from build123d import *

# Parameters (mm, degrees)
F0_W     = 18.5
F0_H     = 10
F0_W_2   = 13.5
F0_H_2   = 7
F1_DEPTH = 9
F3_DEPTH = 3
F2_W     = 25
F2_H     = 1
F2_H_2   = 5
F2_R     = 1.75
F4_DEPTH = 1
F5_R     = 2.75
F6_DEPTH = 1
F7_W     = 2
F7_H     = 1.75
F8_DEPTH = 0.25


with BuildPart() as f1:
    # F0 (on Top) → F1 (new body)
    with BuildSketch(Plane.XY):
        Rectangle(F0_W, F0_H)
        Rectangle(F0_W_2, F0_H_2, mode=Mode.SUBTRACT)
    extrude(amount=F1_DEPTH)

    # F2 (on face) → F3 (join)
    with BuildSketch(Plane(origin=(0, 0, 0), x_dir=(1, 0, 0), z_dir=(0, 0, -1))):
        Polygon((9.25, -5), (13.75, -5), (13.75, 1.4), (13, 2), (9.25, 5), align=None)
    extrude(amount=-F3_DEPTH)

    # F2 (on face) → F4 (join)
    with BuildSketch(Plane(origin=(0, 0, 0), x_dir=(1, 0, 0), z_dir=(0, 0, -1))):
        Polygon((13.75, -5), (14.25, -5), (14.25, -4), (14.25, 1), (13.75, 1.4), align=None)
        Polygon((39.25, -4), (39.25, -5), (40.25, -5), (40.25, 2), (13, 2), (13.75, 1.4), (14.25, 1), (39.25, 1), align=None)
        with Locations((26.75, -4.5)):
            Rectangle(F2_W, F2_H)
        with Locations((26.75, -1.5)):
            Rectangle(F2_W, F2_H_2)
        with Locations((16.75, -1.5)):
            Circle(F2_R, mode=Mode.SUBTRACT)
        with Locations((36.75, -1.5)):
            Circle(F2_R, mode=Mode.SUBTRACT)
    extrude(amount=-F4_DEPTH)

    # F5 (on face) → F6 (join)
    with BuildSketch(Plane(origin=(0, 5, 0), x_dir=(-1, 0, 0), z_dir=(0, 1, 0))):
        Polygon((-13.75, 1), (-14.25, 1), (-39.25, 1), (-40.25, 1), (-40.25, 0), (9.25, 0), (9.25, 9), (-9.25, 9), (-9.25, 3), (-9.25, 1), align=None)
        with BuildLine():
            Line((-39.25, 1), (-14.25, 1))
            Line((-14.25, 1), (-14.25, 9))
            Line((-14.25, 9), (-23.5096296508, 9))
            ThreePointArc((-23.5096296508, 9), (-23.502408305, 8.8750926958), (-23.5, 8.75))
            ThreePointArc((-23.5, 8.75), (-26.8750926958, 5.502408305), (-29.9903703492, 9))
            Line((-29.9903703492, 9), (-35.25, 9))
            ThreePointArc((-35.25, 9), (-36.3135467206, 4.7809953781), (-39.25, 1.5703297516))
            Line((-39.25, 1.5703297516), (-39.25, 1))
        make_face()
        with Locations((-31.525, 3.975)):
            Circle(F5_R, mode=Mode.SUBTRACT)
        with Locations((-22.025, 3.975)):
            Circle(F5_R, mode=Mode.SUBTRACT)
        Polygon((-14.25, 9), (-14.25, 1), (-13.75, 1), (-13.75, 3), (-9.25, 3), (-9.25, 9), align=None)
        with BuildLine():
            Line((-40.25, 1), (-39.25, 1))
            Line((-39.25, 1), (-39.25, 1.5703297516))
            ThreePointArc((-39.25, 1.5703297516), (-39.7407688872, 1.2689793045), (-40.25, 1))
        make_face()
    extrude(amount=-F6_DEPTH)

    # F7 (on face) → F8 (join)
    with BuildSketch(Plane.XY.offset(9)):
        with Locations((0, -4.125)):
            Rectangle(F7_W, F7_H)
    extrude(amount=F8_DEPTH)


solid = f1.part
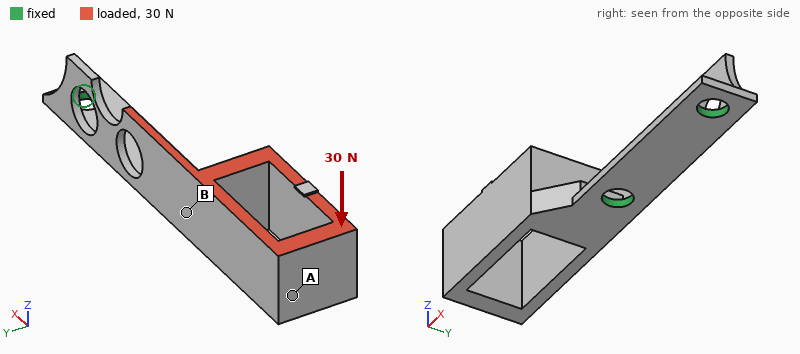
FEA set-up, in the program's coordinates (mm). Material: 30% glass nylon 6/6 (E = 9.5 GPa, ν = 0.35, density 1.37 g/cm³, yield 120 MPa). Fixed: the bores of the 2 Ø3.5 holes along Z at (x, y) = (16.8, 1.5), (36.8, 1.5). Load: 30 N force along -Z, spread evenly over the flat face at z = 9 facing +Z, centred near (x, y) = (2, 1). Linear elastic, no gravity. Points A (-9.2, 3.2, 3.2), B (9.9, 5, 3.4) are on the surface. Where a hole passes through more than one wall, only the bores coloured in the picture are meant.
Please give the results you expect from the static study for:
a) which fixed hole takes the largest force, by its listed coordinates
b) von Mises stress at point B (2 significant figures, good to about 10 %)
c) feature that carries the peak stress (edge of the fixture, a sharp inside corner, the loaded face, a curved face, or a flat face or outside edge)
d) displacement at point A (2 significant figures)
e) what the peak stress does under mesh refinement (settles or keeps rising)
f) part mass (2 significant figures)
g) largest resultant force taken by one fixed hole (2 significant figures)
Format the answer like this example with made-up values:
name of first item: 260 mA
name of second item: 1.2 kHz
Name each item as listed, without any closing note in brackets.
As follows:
which fixed hole takes the largest force, by its listed coordinates: (16.8, 1.5)
von Mises stress at point B: 7.5 MPa
feature that carries the peak stress: edge of the fixture
displacement at point A: 0.33 mm
what the peak stress does under mesh refinement: keeps rising
part mass: 1.7 g
largest resultant force taken by one fixed hole: 48 N
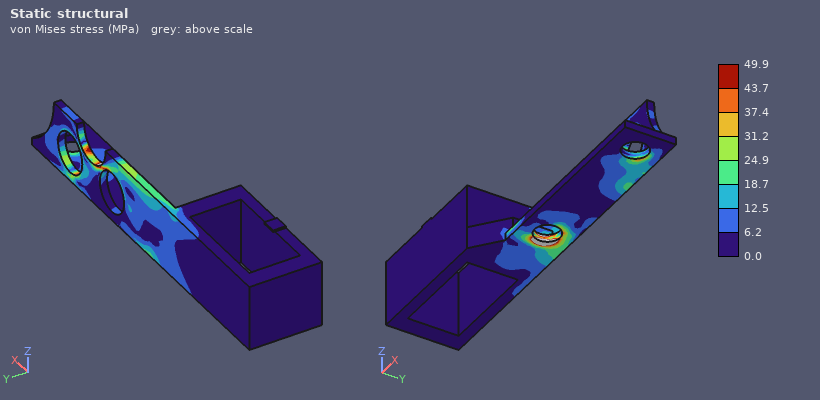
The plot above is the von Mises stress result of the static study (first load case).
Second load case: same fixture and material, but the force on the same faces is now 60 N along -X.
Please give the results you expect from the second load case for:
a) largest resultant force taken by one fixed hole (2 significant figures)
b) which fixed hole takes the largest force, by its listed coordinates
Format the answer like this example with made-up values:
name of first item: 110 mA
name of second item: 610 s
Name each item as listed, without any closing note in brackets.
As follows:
largest resultant force taken by one fixed hole: 39 N
which fixed hole takes the largest force, by its listed coordinates: (16.8, 1.5)
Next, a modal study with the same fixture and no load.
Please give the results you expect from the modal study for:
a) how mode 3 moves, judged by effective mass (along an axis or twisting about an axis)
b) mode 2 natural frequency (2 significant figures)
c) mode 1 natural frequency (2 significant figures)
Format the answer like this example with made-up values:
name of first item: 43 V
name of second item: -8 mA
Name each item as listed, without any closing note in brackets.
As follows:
how mode 3 moves, judged by effective mass: twisting about X
mode 2 natural frequency: 1900 Hz
mode 1 natural frequency: 1400 Hz
